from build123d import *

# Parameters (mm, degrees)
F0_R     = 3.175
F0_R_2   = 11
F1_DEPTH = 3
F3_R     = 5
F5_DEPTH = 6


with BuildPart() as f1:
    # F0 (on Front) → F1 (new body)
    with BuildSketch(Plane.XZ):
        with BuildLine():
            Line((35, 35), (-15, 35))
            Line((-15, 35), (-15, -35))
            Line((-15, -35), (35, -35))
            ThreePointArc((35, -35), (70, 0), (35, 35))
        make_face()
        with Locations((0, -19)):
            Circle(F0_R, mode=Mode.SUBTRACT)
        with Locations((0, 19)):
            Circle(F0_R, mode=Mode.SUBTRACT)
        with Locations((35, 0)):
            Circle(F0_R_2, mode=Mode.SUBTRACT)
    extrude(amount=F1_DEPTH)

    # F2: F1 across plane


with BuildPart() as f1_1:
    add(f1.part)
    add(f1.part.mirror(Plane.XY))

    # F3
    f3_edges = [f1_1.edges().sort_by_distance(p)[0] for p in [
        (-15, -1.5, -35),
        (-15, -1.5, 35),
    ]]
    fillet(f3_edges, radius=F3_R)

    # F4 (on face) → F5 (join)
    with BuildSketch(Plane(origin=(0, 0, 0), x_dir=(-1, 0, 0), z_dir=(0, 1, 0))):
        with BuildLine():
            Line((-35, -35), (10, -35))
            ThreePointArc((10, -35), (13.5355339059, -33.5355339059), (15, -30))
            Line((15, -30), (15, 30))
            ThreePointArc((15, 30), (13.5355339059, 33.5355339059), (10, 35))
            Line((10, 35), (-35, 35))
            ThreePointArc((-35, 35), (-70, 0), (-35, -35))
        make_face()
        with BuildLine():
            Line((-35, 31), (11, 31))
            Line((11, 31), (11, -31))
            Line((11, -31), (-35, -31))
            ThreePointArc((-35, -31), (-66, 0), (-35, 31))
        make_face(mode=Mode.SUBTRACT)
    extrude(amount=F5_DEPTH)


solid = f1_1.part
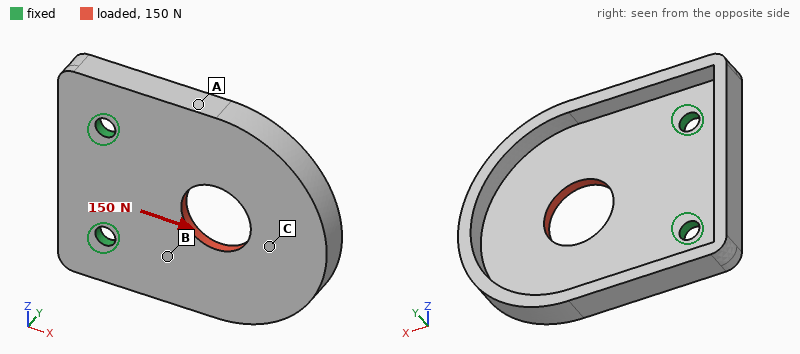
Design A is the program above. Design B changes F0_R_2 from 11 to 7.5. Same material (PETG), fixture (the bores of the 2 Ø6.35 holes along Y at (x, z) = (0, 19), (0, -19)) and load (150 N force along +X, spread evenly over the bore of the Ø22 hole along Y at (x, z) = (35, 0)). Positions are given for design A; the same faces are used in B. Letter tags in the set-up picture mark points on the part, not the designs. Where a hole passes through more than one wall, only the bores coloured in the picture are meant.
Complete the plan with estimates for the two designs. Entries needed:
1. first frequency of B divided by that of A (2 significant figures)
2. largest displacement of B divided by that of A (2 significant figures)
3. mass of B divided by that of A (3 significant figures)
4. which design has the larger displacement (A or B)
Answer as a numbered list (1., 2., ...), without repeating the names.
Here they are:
1. 0.99
2. 0.90
3. 1.03
4. A
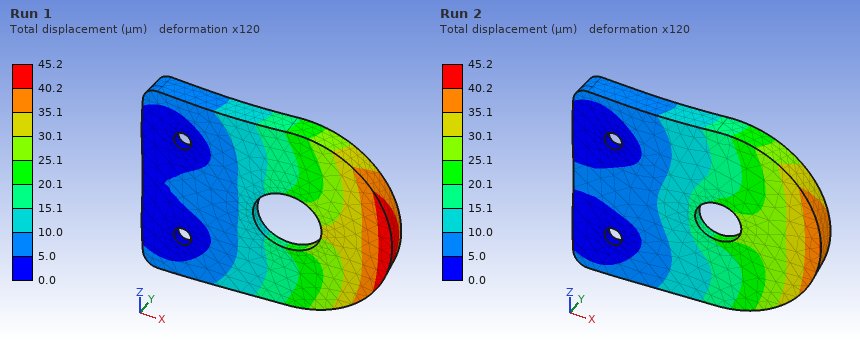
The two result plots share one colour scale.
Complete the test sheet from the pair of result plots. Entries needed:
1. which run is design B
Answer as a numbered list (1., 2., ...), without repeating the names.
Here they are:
1. Run 2
